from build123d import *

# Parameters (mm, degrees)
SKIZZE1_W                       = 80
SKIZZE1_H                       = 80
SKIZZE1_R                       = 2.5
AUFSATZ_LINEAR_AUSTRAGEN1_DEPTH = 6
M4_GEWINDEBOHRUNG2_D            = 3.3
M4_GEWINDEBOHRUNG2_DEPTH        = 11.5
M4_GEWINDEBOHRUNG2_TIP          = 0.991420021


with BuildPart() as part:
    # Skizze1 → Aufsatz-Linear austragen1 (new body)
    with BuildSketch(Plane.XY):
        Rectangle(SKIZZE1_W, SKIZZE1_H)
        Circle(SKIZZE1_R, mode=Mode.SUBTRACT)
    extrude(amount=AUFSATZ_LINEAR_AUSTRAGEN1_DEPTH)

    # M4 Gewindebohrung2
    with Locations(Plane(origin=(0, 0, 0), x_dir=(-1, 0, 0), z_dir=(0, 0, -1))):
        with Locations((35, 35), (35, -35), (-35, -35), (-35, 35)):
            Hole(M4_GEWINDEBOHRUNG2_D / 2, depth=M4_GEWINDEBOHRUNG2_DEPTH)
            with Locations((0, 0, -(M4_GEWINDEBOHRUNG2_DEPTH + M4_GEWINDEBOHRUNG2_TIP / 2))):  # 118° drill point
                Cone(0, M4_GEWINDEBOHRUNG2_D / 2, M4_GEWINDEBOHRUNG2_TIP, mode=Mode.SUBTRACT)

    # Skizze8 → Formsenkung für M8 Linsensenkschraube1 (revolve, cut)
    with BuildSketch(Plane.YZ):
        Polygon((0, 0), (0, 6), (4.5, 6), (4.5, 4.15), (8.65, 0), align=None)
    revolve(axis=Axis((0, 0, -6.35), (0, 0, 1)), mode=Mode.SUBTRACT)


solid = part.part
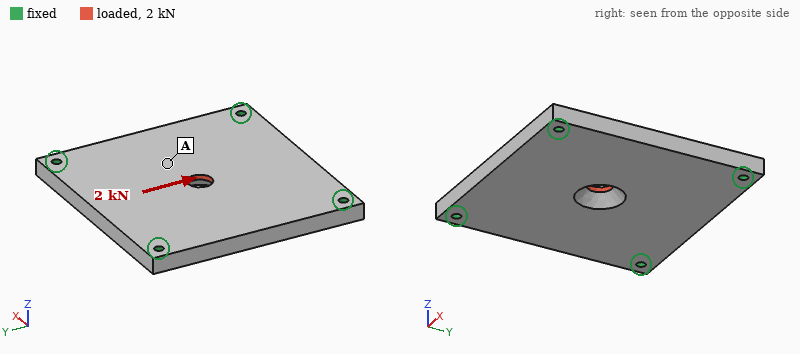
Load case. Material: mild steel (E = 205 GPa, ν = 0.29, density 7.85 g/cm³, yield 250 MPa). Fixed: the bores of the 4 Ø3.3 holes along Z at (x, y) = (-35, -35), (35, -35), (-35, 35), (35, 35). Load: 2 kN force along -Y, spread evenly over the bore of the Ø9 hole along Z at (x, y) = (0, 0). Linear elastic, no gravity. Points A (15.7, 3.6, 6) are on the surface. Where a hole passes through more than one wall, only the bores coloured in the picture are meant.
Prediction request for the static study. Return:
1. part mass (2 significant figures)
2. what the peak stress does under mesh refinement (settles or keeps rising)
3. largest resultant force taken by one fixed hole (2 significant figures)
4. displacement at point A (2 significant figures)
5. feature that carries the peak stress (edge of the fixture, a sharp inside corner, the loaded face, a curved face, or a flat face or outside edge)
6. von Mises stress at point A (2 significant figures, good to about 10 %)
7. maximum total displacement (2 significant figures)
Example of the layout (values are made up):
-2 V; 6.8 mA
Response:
290 g; keeps rising; 570 N; 1.2 µm; a sharp inside corner; 6.4 MPa; 2.6 µm
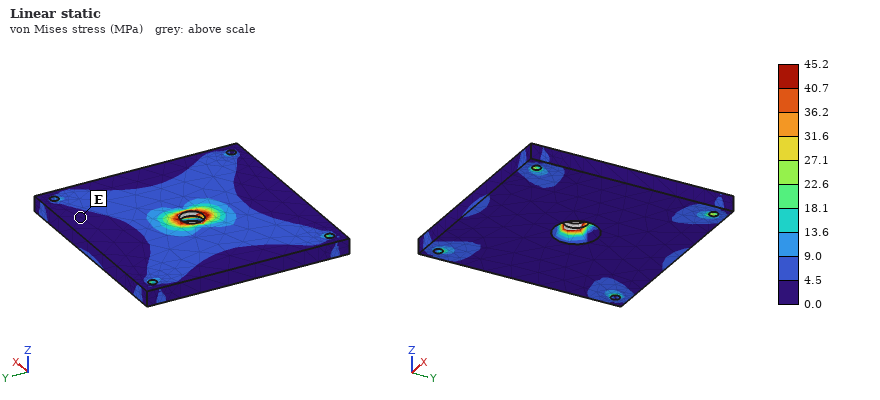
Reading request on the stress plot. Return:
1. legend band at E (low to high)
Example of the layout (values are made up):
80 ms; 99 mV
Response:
0.0 to 4.5 MPa
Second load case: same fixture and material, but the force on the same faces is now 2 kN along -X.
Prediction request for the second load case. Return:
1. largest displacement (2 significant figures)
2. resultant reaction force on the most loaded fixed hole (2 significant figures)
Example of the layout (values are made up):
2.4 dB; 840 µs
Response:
2.6 µm; 570 N
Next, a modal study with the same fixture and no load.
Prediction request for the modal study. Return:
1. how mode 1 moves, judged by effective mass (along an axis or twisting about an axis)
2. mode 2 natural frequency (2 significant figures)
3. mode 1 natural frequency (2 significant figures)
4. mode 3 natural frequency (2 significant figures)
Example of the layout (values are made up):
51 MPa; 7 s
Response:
along Z; 6500 Hz; 3700 Hz; 6500 Hz
